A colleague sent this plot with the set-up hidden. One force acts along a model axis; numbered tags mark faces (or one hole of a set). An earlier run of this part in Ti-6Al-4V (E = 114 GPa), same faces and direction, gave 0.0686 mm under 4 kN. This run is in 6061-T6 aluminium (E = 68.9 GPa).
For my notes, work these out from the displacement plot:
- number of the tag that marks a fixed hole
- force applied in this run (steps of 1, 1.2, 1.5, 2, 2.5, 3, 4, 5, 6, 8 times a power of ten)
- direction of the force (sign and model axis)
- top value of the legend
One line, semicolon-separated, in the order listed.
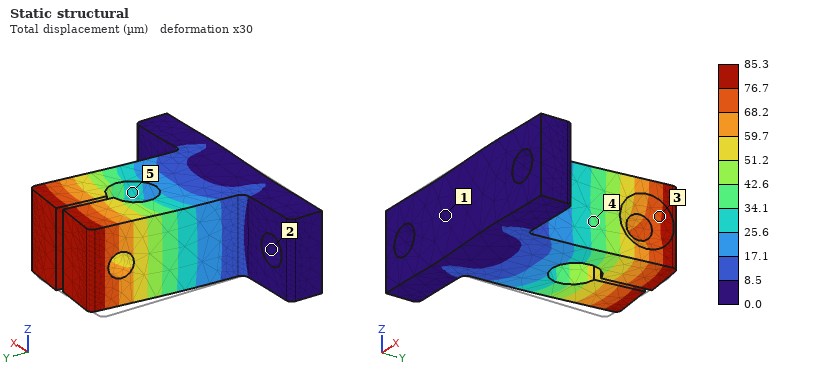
2; 3 kN; +X; 85.3 µm
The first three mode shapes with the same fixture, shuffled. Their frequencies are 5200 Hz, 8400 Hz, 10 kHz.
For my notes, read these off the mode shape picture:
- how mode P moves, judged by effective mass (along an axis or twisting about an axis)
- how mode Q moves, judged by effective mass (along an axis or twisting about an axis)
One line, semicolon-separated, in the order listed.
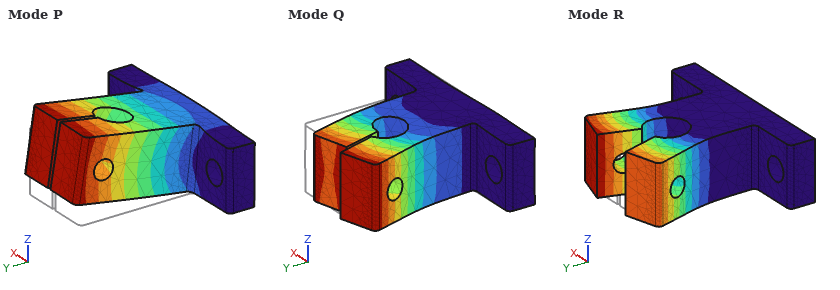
along Z; along X
